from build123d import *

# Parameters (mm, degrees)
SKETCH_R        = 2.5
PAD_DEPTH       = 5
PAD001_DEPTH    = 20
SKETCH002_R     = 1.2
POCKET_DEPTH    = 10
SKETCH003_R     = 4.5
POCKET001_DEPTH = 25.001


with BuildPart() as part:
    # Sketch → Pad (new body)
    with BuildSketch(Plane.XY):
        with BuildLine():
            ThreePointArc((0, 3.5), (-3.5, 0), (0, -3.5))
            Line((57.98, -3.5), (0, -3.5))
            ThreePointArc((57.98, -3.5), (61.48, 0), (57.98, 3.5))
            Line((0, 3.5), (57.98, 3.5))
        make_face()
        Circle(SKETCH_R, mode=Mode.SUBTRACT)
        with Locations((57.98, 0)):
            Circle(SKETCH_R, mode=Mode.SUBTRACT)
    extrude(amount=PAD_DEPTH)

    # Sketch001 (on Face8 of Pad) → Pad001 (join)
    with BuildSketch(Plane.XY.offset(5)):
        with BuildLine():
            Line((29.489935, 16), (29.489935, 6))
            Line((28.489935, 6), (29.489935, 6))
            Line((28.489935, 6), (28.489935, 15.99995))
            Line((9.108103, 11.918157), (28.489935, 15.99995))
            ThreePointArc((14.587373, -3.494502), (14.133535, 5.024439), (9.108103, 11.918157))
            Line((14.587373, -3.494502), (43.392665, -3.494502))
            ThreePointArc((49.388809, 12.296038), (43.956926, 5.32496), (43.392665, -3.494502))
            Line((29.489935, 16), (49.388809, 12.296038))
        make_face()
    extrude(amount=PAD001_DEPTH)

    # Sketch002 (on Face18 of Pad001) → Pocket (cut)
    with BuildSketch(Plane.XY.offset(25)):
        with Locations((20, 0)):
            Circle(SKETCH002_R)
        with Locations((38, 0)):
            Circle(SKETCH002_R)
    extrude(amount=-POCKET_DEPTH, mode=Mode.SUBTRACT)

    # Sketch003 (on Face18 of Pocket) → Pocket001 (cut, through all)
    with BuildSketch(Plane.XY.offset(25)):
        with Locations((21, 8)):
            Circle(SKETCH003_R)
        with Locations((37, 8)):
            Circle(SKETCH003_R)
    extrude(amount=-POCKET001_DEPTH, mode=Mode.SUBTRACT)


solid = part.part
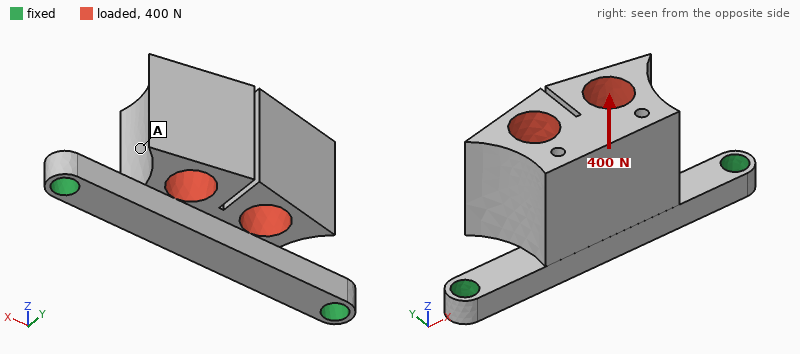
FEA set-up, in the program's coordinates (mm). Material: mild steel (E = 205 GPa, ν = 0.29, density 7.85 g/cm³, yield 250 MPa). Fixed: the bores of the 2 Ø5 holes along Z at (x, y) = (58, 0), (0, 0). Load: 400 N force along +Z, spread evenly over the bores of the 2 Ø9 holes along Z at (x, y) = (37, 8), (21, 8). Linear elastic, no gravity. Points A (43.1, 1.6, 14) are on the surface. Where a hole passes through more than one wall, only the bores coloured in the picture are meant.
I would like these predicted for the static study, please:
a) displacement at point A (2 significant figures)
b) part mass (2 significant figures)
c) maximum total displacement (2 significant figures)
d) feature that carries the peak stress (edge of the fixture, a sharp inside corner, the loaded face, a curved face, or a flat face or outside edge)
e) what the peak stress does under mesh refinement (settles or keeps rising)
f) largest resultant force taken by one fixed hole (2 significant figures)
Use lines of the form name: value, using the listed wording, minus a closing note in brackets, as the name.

displacement at point A: 22 µm
part mass: 82 g
maximum total displacement: 53 µm
feature that carries the peak stress: edge of the fixture
what the peak stress does under mesh refinement: keeps rising
largest resultant force taken by one fixed hole: 230 N
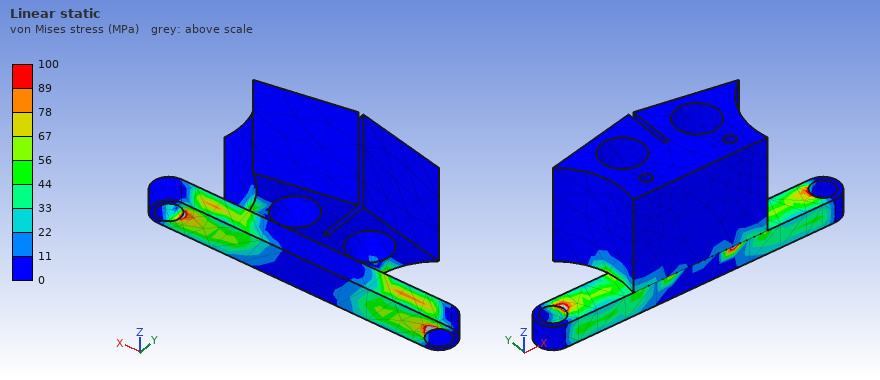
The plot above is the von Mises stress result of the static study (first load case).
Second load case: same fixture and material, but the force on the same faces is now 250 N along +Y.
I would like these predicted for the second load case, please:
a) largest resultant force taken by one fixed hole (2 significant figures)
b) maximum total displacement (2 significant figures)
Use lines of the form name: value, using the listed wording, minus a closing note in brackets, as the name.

largest resultant force taken by one fixed hole: 130 N
maximum total displacement: 51 µm
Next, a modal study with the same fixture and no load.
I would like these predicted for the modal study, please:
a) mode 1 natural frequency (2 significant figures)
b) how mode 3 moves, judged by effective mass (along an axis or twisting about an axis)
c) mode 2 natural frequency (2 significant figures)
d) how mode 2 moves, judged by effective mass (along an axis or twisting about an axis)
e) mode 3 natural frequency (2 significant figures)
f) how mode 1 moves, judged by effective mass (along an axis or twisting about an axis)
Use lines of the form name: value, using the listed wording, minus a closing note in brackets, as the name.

mode 1 natural frequency: 1600 Hz
how mode 3 moves, judged by effective mass: along X
mode 2 natural frequency: 5000 Hz
how mode 2 moves, judged by effective mass: along Z
mode 3 natural frequency: 6000 Hz
how mode 1 moves, judged by effective mass: along Y
